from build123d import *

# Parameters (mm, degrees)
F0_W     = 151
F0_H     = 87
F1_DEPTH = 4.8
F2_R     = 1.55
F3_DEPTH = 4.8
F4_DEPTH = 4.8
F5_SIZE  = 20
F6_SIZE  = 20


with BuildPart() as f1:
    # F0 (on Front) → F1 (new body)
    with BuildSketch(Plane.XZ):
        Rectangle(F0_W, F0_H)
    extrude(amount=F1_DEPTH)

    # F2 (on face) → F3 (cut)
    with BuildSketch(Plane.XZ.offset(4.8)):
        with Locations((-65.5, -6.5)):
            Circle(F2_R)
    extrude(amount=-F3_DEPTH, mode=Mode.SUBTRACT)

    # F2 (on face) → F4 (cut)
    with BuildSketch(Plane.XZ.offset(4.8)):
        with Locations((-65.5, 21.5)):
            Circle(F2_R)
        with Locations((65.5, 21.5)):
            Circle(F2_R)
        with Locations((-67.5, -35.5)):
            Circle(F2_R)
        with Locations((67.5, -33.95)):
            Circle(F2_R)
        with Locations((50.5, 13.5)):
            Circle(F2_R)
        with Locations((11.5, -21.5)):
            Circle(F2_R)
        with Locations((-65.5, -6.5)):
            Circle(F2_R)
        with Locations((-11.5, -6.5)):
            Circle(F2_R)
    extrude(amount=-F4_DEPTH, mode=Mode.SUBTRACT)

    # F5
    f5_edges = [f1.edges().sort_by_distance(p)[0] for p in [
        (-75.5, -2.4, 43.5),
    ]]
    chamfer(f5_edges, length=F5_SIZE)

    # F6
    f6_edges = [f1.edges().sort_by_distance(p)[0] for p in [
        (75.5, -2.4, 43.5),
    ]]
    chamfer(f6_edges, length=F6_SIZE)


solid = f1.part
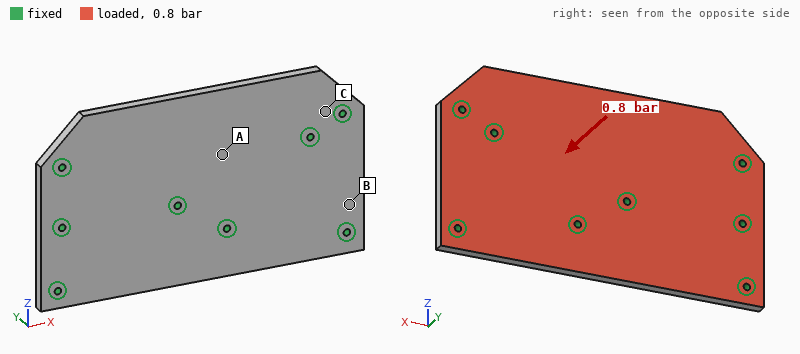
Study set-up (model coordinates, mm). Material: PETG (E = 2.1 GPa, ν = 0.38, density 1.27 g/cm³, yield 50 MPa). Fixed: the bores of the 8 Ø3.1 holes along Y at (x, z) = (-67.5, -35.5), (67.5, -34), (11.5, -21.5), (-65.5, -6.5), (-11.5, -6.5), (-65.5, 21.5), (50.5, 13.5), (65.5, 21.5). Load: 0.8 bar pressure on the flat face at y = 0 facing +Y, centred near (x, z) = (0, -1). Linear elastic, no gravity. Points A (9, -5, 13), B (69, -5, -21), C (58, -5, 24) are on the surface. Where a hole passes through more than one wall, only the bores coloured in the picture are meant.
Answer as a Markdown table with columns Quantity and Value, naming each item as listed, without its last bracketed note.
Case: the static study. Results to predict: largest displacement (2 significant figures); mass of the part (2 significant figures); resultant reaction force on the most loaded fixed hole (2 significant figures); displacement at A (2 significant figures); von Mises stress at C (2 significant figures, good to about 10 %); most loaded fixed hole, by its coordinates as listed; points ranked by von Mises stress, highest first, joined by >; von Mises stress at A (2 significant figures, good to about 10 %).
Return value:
| Quantity | Value |
|---|---|
| largest displacement | 1.8 mm |
| mass of the part | 77 g |
| resultant reaction force on the most loaded fixed hole | 280 N |
| displacement at A | 0.59 mm |
| von Mises stress at C | 9.1 MPa |
| most loaded fixed hole, by its coordinates as listed | (-11.5, -6.5) |
| points ranked by von Mises stress, highest first, joined by > | C > A > B |
| von Mises stress at A | 5.3 MPa |
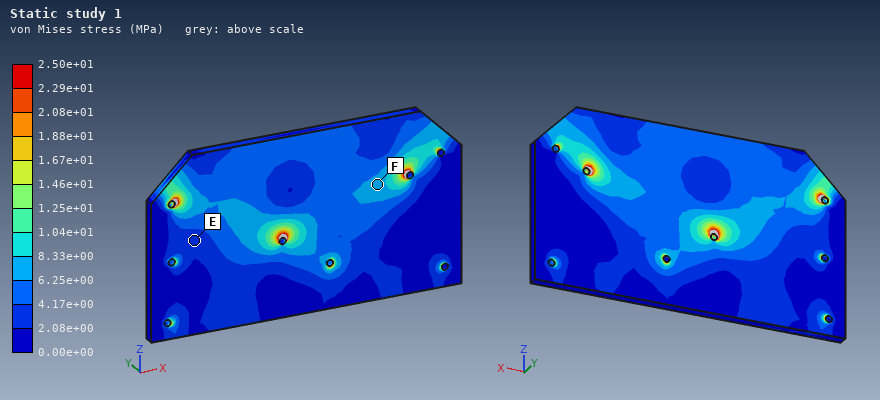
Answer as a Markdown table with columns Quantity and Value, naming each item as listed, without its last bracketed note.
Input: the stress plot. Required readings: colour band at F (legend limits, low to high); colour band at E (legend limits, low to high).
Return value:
| Quantity | Value |
|---|---|
| colour band at F | 6.25e+00 to 8.33e+00 MPa |
| colour band at E | 2.08e+00 to 4.17e+00 MPa |
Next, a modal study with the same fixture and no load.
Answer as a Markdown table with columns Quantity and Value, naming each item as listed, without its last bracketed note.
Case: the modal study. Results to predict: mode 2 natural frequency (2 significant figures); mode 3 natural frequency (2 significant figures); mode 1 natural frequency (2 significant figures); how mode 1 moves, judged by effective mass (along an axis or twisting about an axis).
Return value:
| Quantity | Value |
|---|---|
| mode 2 natural frequency | 1100 Hz |
| mode 3 natural frequency | 1100 Hz |
| mode 1 natural frequency | 570 Hz |
| how mode 1 moves, judged by effective mass | along Y |
